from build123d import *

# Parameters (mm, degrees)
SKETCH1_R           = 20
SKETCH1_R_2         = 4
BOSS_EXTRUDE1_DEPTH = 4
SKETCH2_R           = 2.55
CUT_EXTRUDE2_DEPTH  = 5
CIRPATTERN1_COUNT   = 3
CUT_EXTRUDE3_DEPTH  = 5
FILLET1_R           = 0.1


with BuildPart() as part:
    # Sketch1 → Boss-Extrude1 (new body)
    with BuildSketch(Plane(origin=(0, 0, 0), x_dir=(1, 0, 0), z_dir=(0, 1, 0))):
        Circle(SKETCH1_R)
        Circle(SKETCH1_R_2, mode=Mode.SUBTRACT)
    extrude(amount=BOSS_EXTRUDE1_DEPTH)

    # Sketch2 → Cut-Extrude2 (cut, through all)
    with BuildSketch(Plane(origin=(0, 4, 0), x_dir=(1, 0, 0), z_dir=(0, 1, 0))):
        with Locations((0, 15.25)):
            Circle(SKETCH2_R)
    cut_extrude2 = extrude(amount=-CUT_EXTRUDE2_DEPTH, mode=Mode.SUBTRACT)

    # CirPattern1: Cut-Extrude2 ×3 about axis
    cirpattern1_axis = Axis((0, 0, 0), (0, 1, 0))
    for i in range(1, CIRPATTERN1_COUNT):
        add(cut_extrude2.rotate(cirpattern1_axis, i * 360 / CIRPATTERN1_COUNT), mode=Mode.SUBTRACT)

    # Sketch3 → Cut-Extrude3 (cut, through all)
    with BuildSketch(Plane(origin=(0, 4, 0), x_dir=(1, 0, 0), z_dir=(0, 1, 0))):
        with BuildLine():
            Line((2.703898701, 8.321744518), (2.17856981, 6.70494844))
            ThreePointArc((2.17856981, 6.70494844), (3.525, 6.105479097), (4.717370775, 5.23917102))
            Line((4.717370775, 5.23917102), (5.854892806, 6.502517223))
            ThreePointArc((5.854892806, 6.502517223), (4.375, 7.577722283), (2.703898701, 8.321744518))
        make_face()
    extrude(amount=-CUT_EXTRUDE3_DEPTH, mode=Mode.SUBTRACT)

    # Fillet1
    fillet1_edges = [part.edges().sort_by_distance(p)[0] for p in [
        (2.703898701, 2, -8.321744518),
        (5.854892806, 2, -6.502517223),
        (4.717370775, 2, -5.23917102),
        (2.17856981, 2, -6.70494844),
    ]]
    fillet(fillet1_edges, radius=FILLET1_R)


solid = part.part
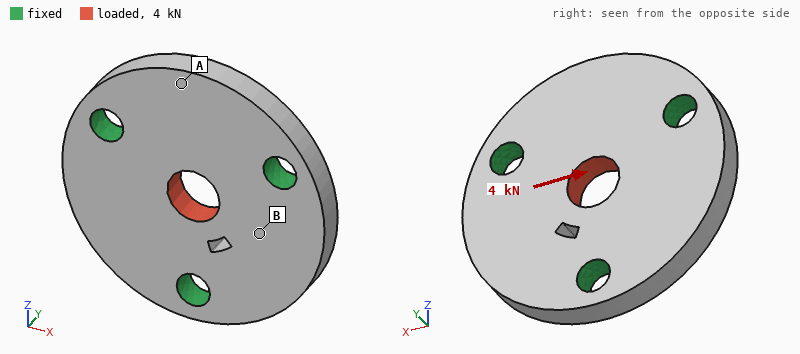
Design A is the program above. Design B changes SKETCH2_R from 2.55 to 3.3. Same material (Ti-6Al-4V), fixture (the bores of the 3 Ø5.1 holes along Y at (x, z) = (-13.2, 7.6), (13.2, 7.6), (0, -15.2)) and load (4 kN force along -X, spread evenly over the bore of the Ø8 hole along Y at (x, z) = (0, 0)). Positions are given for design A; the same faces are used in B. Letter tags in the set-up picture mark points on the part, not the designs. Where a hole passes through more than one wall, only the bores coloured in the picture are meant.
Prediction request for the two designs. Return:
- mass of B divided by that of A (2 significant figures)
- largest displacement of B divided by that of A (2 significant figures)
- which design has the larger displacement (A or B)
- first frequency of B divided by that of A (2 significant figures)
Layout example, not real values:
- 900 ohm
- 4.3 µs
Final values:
- 0.96
- 0.92
- A
- 1.1
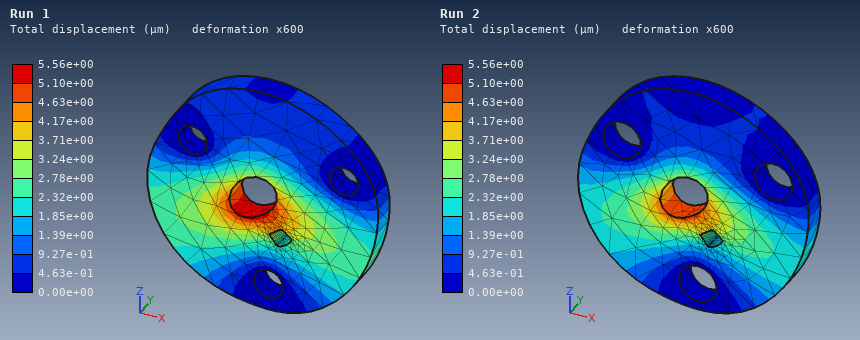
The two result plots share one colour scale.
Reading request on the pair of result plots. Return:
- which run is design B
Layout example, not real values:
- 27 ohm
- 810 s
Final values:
- Run 2
